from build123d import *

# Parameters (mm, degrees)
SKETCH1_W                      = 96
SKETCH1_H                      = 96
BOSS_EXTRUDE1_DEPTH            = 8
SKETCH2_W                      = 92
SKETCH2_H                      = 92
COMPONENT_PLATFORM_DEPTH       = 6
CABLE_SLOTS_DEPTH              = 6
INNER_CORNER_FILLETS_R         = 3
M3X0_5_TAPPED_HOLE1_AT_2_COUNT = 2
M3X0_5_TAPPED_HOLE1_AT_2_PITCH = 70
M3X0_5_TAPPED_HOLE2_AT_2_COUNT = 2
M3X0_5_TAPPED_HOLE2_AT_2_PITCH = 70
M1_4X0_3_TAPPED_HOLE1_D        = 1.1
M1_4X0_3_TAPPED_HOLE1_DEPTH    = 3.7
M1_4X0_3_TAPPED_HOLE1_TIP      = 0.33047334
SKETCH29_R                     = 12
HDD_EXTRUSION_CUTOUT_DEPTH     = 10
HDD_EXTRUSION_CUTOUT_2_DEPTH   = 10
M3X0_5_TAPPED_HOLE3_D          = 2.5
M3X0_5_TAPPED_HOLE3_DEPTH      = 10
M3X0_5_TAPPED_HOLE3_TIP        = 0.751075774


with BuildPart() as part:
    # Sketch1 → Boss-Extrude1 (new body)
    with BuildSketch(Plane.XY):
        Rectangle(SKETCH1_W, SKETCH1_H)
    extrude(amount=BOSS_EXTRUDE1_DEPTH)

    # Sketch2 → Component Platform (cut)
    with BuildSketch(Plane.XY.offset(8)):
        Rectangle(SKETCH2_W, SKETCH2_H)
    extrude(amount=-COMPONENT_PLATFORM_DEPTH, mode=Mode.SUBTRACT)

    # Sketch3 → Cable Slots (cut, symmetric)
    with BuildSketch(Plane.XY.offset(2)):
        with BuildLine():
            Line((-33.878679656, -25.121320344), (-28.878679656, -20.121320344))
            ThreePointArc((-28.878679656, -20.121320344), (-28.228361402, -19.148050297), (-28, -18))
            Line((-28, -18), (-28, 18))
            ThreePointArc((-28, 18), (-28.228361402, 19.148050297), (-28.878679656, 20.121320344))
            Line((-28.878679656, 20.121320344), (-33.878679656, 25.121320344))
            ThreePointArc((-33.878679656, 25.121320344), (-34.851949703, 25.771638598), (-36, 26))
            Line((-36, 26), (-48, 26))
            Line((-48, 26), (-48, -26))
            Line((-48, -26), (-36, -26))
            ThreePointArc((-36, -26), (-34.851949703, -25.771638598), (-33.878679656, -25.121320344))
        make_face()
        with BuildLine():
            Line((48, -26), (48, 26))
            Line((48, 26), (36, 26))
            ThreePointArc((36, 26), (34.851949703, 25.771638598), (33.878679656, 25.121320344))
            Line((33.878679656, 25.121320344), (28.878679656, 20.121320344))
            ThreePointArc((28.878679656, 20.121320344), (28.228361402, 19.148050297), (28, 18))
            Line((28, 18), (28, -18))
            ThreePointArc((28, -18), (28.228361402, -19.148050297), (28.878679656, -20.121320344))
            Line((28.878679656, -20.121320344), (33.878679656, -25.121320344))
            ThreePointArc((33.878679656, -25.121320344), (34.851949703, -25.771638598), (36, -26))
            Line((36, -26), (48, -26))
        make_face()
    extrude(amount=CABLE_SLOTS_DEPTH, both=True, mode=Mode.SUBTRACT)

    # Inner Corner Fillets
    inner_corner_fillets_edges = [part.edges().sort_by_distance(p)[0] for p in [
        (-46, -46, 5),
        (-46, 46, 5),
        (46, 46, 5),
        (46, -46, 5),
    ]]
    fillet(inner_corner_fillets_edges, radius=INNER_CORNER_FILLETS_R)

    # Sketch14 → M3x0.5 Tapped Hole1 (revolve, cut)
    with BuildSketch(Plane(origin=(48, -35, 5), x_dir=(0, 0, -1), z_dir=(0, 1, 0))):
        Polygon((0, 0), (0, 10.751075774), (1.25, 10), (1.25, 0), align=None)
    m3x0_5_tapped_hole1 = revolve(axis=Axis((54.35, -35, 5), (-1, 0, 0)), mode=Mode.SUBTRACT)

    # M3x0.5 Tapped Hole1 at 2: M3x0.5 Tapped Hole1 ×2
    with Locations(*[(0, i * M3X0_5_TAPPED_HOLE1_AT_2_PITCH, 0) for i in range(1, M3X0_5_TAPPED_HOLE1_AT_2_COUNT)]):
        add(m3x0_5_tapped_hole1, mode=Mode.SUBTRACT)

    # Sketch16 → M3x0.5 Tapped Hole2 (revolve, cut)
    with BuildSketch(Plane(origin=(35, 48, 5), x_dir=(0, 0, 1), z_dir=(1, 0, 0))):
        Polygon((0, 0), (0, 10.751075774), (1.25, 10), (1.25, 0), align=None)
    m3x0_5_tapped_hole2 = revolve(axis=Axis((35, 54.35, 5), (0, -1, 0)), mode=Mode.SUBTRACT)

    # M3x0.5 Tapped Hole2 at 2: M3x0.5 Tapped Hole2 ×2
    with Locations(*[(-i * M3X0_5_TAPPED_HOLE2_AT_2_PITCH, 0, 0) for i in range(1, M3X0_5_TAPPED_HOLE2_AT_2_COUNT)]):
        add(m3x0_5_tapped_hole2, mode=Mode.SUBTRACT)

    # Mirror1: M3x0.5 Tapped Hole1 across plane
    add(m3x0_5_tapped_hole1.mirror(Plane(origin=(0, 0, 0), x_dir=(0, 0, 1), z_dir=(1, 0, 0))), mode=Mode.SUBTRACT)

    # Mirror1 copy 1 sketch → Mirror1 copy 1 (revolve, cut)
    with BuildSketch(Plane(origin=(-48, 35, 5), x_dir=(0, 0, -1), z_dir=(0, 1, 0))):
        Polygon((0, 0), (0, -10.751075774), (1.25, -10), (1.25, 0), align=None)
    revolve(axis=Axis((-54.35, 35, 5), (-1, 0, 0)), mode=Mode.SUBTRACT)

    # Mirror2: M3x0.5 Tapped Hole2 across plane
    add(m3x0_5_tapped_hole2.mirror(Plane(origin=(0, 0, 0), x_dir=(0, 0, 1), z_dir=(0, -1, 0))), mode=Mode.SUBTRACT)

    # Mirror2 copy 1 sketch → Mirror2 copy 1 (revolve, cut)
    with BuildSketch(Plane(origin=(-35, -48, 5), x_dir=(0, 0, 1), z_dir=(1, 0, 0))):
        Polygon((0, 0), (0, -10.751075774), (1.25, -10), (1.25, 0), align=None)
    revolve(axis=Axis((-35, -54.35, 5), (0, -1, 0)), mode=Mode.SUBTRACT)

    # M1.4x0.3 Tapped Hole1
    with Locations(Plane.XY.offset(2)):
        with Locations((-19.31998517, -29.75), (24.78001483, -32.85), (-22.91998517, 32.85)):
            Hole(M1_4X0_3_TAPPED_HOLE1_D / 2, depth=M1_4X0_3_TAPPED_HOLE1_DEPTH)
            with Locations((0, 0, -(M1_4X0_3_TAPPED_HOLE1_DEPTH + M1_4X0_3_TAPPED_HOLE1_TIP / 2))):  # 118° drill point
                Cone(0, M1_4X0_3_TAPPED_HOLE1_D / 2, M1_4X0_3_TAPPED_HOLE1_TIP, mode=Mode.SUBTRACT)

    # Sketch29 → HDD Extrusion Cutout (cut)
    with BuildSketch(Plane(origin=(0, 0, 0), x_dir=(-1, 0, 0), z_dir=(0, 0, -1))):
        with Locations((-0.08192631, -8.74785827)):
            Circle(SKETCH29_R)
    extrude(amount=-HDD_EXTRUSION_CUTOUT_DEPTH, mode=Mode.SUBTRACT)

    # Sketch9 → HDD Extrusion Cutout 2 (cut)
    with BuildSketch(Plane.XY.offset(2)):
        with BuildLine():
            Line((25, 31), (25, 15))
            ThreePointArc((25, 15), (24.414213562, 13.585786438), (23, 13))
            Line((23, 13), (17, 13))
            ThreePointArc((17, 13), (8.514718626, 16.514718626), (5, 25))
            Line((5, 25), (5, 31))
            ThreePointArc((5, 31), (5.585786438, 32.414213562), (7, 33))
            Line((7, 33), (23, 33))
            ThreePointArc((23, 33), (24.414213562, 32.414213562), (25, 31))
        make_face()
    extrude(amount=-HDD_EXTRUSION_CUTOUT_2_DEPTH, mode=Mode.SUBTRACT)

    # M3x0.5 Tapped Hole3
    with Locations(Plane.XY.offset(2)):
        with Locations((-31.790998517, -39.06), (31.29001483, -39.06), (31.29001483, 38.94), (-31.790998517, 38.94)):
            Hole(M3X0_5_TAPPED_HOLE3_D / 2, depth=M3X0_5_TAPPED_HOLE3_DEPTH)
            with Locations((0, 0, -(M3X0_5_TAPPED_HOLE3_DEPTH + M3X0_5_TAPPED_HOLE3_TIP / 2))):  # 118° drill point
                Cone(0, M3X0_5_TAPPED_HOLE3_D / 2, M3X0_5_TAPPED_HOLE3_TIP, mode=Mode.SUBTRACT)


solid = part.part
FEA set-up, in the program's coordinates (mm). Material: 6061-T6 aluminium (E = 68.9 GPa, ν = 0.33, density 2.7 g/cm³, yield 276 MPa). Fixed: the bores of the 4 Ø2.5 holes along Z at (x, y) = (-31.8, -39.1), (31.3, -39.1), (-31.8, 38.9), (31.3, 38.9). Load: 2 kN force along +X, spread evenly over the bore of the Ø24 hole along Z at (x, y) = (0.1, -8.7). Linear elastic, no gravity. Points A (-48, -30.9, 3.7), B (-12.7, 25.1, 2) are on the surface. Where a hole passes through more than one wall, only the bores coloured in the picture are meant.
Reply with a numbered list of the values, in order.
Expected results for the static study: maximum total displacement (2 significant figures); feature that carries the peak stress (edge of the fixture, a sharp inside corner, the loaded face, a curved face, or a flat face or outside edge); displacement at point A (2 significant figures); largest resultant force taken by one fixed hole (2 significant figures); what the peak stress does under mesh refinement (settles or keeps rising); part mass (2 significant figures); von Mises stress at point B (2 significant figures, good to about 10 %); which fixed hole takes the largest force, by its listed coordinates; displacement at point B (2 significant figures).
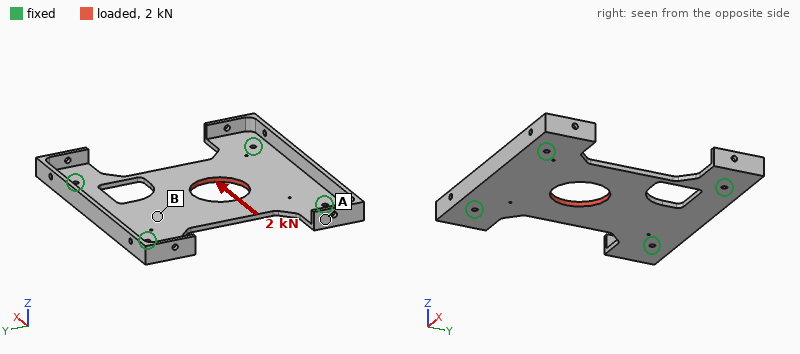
1. 23 µm
2. edge of the fixture
3. 11 µm
4. 860 N
5. keeps rising
6. 43 g
7. 15 MPa
8. (-31.8, -39.1)
9. 9.7 µm
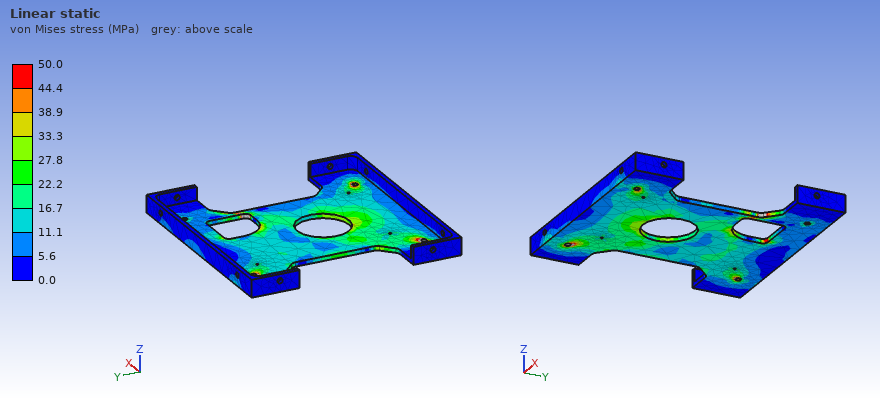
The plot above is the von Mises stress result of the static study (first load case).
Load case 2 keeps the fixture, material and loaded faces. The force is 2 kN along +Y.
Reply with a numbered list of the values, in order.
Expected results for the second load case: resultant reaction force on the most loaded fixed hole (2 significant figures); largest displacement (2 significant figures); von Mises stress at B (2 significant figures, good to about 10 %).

1. 720 N
2. 21 µm
3. 5.1 MPa
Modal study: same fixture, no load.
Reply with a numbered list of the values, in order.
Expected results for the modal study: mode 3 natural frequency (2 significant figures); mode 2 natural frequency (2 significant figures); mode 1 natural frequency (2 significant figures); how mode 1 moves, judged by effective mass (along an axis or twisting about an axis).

1. 3100 Hz
2. 2400 Hz
3. 1400 Hz
4. along Z
